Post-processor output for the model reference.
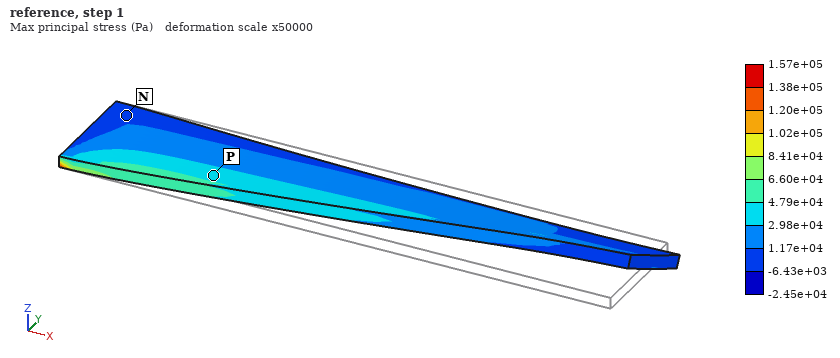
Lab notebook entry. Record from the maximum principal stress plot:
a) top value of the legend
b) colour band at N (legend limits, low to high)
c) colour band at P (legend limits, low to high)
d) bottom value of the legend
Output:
1.57e+05 Pa
-6.43e+03 to 1.17e+04 Pa
2.98e+04 to 4.79e+04 Pa
-2.45e+04 Pa
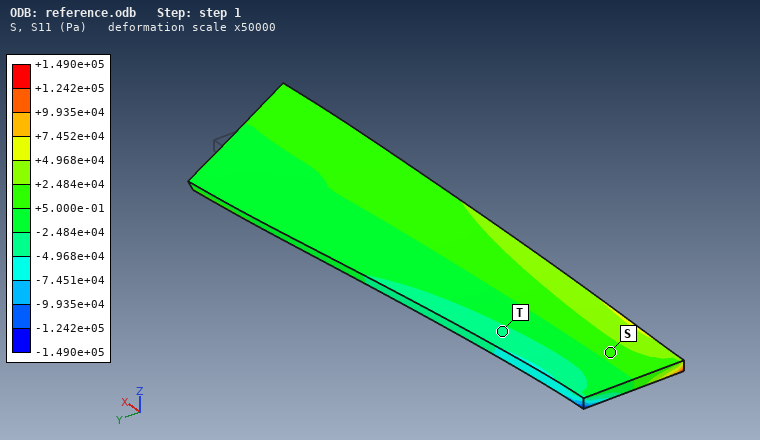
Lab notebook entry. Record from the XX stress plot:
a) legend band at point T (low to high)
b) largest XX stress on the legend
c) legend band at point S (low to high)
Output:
-4.968e+04 to -2.484e+04 Pa
+1.490e+05 Pa
+5.000e-01 to +2.484e+04 Pa
